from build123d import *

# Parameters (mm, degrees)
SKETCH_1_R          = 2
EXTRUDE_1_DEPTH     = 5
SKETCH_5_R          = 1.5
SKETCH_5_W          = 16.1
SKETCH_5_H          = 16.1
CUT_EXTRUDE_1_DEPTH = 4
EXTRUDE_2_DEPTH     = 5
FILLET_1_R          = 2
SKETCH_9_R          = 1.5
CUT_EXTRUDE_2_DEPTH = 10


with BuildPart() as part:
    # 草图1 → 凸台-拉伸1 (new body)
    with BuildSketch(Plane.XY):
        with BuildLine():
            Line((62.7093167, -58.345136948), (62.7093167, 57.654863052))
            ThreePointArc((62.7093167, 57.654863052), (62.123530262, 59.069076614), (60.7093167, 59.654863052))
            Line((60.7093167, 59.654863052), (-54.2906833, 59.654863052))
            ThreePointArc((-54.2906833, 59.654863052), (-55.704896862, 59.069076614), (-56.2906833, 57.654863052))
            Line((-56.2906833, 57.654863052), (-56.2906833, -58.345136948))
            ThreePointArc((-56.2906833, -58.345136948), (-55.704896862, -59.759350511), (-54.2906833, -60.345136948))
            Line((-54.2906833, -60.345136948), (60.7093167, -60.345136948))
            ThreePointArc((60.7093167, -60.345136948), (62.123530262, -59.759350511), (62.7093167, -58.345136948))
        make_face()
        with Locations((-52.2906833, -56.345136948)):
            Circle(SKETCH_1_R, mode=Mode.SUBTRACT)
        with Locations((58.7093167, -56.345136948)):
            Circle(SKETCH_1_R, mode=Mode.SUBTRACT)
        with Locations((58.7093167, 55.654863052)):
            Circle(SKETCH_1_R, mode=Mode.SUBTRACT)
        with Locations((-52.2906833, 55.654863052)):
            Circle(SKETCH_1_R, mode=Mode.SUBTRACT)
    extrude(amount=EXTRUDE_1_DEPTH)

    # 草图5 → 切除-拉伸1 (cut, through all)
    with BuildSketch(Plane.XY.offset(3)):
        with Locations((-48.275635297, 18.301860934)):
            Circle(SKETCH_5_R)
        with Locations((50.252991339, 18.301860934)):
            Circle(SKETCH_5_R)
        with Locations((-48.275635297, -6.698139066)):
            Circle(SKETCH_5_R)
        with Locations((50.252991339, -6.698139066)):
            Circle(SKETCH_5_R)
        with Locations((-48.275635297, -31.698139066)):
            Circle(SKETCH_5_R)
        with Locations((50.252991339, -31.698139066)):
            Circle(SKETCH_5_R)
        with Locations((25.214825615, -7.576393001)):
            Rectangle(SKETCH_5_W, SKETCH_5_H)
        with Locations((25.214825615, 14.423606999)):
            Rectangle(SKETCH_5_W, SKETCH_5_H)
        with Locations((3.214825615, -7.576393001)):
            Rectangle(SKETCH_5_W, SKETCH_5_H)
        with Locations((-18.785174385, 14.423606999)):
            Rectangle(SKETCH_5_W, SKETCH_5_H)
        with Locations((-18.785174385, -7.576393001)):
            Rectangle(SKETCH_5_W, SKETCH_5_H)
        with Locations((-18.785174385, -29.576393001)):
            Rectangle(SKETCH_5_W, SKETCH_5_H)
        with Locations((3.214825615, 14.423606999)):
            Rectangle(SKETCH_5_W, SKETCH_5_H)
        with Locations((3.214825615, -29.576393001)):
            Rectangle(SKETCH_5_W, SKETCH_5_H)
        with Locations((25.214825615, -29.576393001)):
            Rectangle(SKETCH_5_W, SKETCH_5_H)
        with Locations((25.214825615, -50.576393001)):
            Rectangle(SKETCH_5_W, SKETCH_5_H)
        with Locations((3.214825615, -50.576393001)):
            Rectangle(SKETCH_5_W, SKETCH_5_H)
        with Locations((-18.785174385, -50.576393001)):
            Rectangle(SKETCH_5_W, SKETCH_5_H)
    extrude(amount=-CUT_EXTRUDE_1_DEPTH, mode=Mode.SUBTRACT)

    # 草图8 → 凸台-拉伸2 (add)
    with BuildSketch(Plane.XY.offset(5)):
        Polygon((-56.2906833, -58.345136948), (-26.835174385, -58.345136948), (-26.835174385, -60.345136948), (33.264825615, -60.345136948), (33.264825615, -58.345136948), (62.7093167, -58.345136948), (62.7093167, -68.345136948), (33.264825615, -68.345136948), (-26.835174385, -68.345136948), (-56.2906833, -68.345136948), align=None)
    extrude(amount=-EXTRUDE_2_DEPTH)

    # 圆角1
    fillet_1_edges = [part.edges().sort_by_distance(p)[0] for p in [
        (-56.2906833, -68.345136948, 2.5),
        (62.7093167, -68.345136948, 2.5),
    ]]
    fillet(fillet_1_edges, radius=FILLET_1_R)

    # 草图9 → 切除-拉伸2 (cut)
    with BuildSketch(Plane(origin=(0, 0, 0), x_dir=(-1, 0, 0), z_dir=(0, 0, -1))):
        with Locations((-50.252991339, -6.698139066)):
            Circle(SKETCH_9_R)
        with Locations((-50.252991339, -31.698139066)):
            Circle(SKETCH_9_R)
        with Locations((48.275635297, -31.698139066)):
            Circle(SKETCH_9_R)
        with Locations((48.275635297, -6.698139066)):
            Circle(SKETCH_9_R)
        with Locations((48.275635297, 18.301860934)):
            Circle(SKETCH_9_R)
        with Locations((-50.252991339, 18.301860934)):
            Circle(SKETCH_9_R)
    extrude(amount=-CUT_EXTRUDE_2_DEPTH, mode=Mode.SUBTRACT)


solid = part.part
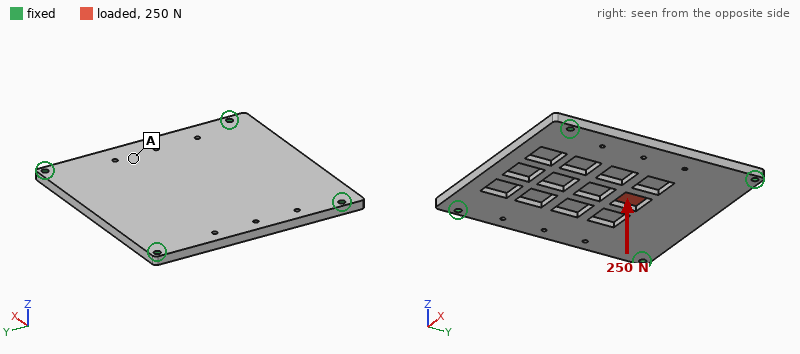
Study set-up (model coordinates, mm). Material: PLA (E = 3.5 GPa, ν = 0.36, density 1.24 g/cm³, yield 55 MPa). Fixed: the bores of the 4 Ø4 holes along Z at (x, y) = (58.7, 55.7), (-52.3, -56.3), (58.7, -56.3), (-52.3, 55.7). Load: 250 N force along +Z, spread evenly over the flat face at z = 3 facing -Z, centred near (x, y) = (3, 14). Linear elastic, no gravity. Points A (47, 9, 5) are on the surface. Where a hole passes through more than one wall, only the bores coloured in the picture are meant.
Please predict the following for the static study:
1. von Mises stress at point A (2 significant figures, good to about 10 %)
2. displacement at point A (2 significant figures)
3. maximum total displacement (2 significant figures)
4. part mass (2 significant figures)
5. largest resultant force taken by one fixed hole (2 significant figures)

6.0 MPa
0.80 mm
1.9 mm
82 g
120 N
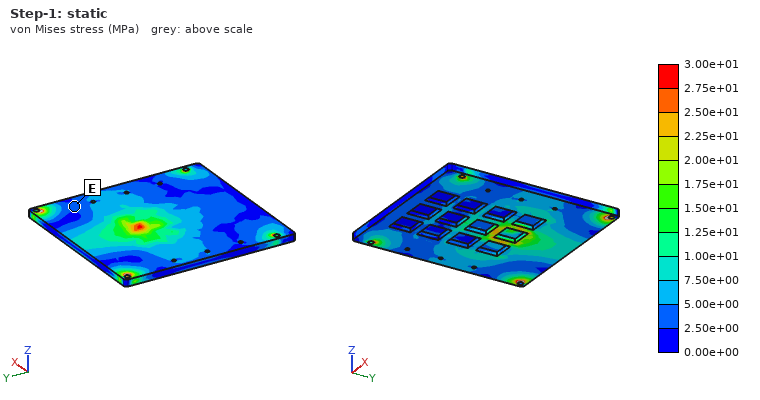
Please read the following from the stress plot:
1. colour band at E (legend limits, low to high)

2.50e+00 to 5.00e+00 MPa
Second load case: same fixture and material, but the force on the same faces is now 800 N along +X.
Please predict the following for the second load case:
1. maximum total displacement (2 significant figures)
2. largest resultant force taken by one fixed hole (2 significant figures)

86 µm
290 N
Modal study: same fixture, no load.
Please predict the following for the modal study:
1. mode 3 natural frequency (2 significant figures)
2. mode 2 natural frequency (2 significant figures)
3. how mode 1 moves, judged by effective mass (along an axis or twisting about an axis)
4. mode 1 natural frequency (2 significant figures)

720 Hz
700 Hz
along Z
410 Hz
